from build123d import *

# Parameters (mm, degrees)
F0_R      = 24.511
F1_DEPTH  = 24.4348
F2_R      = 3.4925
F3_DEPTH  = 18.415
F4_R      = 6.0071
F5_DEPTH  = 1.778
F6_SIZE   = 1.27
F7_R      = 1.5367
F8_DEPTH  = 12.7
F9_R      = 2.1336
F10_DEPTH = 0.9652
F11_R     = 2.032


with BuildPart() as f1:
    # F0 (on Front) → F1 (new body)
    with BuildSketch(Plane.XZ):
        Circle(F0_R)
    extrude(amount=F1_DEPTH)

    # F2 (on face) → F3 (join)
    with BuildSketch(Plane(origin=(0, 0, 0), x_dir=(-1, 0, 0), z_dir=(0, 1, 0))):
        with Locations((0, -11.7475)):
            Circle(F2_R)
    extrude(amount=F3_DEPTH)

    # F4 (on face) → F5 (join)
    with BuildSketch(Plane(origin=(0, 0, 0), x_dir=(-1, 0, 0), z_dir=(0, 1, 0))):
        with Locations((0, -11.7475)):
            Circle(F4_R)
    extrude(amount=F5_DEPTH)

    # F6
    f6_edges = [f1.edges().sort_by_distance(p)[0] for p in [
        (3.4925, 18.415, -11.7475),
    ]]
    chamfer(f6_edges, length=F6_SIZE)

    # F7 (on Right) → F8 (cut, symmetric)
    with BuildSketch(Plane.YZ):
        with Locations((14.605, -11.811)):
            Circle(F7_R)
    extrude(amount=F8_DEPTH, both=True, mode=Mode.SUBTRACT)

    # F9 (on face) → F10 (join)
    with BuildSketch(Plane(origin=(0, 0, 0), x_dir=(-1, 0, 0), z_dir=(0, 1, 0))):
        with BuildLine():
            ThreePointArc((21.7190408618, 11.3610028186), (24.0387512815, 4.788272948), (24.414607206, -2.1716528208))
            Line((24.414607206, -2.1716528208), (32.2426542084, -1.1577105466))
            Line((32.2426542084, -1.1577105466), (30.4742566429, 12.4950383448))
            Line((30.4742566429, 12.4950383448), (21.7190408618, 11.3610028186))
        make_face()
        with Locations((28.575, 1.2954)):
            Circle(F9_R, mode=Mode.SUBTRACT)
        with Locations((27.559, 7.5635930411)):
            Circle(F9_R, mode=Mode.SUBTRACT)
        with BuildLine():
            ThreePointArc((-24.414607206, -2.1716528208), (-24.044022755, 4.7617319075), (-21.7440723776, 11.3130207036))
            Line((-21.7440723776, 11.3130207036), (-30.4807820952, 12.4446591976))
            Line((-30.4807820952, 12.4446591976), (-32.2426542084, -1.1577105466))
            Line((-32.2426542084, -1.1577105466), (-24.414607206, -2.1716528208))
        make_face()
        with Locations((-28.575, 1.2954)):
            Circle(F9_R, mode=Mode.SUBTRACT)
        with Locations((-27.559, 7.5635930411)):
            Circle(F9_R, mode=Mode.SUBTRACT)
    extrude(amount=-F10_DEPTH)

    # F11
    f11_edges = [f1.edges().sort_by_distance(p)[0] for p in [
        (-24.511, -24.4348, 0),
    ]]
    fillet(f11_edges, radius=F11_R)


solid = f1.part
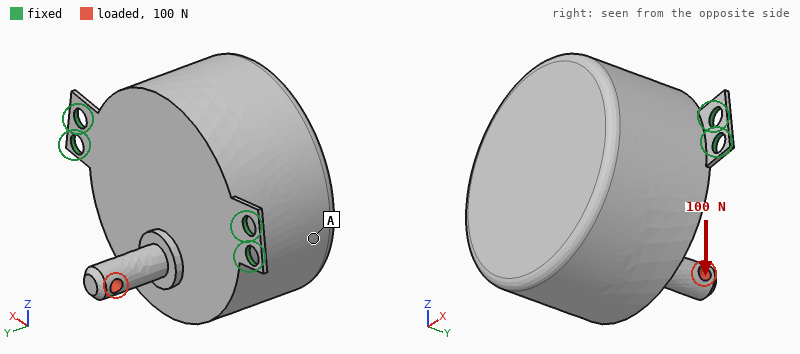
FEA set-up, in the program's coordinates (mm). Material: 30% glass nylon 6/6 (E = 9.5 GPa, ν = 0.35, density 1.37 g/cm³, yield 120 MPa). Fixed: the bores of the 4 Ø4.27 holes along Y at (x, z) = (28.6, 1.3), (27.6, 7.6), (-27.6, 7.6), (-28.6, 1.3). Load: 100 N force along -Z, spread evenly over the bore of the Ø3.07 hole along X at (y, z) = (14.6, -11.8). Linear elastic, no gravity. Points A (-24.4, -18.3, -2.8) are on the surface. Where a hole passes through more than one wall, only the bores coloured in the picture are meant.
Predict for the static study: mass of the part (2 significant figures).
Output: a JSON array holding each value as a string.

["64 g"]
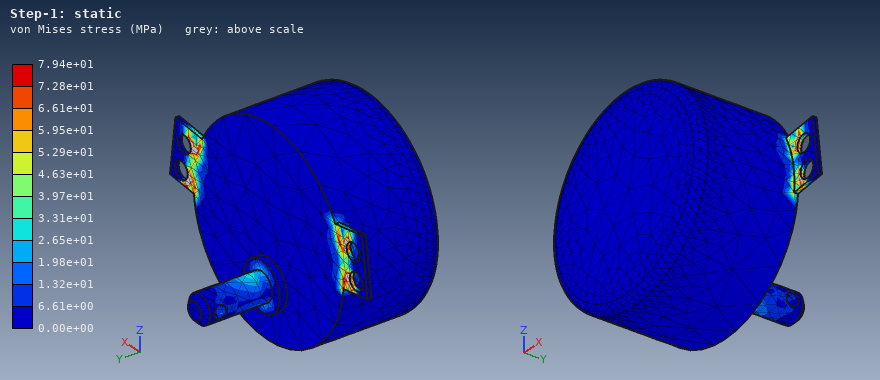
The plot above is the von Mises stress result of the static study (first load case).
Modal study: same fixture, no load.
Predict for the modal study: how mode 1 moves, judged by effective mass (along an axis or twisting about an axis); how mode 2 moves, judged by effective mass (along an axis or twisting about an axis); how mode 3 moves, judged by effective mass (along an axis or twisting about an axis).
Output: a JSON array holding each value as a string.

["along Z", "along Y", "along X"]
